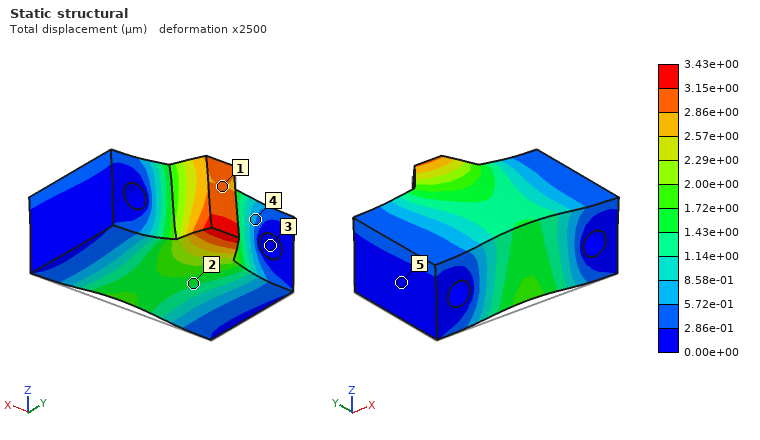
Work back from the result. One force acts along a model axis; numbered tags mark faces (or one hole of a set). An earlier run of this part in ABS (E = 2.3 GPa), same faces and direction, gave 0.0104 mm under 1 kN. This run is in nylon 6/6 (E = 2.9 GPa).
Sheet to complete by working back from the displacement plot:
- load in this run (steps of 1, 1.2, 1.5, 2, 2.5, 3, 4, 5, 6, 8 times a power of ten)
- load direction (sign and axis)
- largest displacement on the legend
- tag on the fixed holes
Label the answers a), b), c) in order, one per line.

a) 400 N
b) +Z
c) 3.43e+00 µm
d) 3
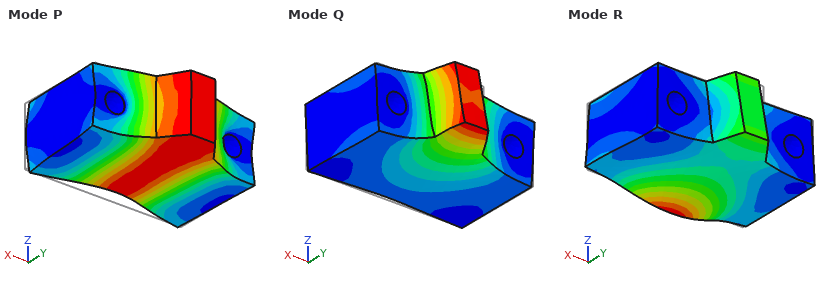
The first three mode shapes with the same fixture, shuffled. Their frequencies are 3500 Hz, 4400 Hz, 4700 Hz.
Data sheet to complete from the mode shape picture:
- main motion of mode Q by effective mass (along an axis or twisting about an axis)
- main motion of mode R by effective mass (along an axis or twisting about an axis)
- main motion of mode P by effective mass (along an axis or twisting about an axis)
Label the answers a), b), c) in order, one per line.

a) along Z
b) along Z
c) along Y
